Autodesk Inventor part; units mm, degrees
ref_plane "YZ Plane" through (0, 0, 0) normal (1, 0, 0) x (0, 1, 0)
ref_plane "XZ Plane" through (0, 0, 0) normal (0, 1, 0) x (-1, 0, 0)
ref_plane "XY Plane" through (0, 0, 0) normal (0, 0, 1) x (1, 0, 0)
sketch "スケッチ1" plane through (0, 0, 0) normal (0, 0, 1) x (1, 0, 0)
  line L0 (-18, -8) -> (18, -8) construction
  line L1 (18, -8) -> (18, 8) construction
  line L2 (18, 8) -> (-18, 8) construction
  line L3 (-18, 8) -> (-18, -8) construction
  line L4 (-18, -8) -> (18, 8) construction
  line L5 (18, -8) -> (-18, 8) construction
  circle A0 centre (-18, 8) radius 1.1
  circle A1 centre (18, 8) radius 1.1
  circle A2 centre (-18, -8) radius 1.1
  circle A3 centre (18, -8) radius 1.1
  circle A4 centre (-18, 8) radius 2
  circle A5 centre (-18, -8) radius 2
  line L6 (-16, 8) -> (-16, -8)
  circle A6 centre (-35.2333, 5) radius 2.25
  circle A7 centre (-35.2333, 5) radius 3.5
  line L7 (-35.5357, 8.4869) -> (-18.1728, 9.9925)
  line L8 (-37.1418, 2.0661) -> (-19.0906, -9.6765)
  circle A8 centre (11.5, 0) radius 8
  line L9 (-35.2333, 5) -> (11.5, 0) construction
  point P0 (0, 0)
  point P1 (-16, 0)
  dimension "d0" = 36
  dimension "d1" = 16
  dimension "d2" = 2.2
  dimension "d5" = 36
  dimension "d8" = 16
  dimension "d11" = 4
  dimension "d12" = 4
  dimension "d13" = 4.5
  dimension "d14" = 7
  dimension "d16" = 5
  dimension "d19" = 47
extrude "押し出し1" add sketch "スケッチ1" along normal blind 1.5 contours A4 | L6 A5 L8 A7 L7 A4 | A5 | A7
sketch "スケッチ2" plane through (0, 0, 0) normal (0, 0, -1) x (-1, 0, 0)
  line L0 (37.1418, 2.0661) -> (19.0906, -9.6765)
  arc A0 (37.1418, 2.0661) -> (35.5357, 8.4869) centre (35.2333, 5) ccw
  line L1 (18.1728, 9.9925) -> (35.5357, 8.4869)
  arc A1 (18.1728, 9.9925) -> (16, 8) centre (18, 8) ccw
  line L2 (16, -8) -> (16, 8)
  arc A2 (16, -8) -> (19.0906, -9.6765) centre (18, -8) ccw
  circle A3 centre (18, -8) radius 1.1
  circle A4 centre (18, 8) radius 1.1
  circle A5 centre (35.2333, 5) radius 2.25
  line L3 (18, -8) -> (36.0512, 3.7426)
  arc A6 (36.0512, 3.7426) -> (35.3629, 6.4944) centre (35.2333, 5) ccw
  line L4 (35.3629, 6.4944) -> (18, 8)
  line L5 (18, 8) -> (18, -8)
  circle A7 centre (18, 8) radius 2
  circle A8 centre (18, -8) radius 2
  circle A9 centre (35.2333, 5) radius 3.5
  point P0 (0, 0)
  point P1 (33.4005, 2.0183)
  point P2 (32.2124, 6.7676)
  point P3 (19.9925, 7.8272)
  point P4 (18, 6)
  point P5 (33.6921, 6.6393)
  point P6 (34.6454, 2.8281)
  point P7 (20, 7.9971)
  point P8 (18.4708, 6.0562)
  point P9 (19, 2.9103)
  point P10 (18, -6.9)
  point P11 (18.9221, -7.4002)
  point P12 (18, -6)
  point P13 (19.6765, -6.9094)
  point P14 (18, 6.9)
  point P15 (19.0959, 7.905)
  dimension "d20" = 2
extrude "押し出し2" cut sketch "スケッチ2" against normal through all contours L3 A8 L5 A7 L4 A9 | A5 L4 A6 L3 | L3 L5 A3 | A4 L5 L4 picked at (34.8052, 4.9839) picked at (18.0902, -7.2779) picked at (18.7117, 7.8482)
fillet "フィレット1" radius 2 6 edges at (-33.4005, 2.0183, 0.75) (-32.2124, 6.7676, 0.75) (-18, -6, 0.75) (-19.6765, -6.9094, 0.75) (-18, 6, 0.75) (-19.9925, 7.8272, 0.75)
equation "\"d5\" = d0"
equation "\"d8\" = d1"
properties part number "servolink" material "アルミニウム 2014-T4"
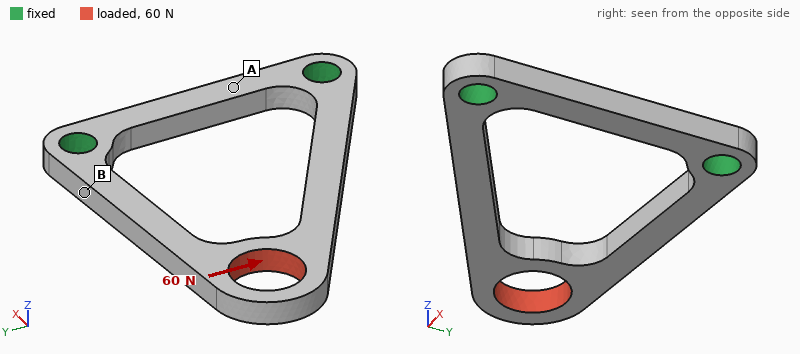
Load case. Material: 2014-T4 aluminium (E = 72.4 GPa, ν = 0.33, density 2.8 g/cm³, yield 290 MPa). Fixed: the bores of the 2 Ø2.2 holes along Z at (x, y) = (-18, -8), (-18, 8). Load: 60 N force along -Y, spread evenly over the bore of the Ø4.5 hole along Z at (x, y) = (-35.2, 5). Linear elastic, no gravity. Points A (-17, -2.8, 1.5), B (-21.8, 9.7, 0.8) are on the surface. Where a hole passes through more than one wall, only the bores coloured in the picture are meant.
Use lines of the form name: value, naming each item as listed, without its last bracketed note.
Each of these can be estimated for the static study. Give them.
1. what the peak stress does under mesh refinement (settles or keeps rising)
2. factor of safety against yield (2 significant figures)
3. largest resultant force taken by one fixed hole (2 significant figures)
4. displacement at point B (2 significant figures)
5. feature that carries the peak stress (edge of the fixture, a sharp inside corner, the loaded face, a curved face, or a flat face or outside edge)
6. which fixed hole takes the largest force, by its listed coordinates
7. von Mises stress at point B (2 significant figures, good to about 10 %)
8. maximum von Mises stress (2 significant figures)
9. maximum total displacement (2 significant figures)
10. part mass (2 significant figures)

what the peak stress does under mesh refinement: settles
factor of safety against yield: 2.5
largest resultant force taken by one fixed hole: 61 N
displacement at point B: 5.6 µm
feature that carries the peak stress: a curved face
which fixed hole takes the largest force, by its listed coordinates: (-18, -8)
von Mises stress at point B: 75 MPa
maximum von Mises stress: 110 MPa
maximum total displacement: 37 µm
part mass: 0.55 g
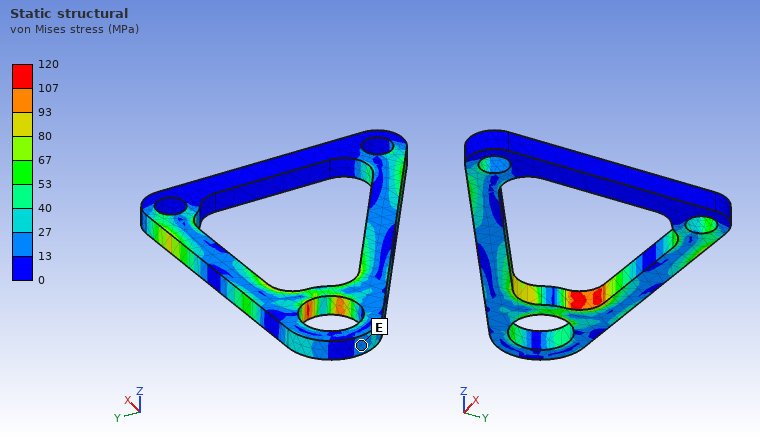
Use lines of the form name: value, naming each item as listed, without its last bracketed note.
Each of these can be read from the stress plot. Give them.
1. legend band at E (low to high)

legend band at E: 13 to 27 MPa
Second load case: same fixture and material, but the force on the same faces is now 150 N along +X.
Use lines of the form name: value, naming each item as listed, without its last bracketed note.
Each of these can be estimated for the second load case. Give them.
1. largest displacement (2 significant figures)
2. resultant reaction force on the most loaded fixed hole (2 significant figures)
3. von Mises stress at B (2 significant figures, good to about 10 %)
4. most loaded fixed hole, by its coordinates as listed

largest displacement: 24 µm
resultant reaction force on the most loaded fixed hole: 110 N
von Mises stress at B: 67 MPa
most loaded fixed hole, by its coordinates as listed: (-18, 8)
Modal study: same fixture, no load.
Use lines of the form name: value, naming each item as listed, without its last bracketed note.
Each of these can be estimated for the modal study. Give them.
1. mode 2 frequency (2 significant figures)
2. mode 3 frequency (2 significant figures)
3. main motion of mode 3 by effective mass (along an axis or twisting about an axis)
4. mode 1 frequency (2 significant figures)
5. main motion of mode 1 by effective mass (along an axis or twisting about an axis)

mode 2 frequency: 11 kHz
mode 3 frequency: 13 kHz
main motion of mode 3 by effective mass: along Y
mode 1 frequency: 2900 Hz
main motion of mode 1 by effective mass: along Z
